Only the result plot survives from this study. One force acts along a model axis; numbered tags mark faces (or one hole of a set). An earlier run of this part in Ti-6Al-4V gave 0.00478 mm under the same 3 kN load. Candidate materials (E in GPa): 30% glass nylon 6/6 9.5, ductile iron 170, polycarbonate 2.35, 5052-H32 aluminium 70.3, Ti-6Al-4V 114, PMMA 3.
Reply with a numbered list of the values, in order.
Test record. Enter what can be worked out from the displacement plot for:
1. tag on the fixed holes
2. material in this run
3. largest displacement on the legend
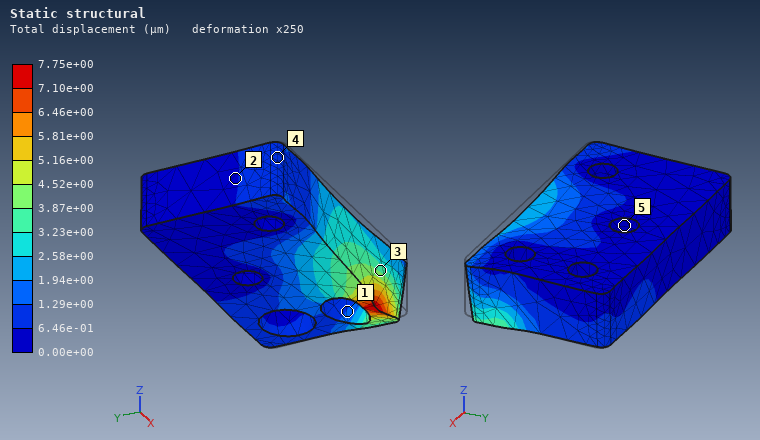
1. 5
2. 5052-H32 aluminium
3. 7.75e+00 µm
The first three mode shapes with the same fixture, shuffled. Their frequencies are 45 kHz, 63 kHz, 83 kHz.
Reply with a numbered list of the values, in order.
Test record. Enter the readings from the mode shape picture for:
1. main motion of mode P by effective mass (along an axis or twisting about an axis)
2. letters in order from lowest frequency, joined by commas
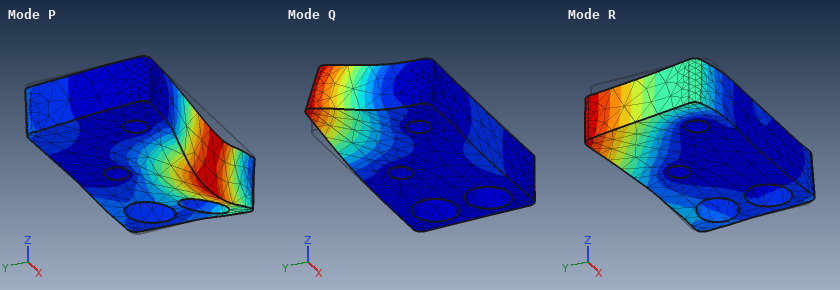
1. along Z
2. Q, P, R
